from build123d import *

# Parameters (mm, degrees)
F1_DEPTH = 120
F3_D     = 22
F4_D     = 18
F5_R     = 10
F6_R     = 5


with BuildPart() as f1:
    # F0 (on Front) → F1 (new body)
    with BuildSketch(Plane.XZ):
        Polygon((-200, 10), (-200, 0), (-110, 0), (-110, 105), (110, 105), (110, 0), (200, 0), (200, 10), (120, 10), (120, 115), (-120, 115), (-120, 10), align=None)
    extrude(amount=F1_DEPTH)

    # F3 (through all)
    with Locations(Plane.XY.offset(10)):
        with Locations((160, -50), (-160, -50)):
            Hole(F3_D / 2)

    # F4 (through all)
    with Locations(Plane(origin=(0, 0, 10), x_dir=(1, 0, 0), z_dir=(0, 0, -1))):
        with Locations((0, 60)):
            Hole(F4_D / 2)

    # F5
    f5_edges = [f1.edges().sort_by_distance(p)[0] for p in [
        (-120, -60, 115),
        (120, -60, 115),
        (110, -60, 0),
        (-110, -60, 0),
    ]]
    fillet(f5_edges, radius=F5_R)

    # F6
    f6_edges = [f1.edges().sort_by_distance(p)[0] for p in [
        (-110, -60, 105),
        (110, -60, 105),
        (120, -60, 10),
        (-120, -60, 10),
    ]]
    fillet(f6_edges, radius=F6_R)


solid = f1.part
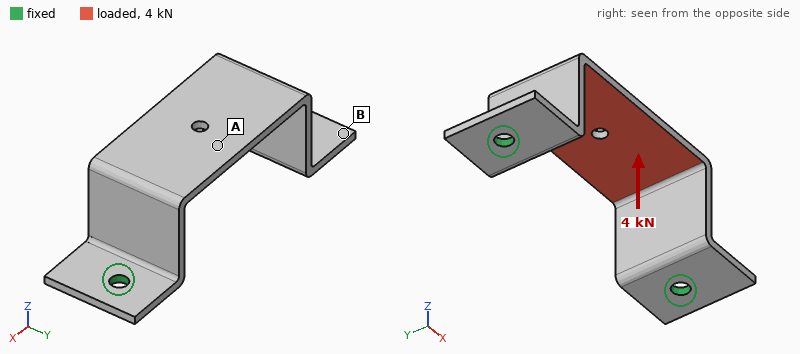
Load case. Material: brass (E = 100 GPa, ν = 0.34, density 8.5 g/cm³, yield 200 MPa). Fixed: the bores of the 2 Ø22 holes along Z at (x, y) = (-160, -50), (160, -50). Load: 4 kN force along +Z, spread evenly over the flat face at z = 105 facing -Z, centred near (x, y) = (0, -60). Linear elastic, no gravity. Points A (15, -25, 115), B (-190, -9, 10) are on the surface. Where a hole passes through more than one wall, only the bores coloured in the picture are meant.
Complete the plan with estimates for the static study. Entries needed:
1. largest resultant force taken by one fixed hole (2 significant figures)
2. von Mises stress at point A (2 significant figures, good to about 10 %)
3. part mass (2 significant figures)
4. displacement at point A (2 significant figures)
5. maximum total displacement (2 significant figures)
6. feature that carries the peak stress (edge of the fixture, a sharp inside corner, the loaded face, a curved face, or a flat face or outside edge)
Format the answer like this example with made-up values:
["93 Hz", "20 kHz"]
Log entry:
["2.3 kN", "26 MPa", "6.1 kg", "0.21 mm", "0.26 mm", "a curved face"]
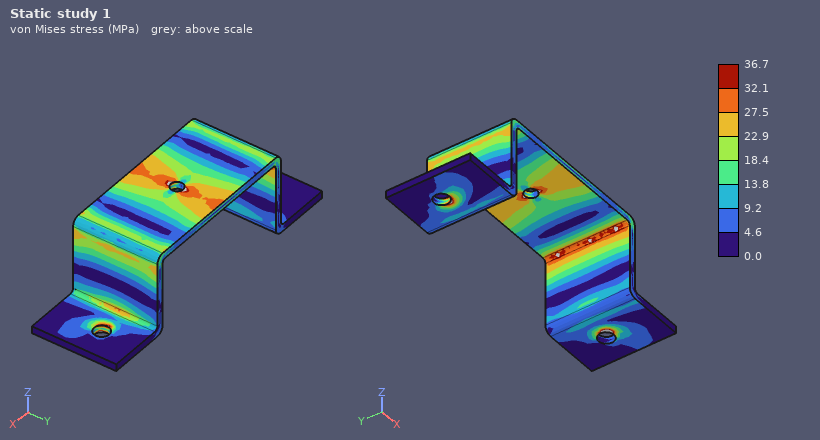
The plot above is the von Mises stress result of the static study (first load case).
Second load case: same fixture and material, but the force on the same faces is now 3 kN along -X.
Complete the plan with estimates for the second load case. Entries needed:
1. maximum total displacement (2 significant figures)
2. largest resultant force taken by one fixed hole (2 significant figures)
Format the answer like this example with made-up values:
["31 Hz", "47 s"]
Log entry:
["0.37 mm", "1.6 kN"]
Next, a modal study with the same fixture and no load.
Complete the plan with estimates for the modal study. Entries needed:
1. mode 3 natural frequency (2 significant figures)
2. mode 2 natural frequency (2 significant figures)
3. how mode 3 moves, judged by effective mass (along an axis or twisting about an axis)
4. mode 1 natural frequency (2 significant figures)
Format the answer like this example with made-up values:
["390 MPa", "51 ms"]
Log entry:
["390 Hz", "260 Hz", "twisting about Z", "250 Hz"]
